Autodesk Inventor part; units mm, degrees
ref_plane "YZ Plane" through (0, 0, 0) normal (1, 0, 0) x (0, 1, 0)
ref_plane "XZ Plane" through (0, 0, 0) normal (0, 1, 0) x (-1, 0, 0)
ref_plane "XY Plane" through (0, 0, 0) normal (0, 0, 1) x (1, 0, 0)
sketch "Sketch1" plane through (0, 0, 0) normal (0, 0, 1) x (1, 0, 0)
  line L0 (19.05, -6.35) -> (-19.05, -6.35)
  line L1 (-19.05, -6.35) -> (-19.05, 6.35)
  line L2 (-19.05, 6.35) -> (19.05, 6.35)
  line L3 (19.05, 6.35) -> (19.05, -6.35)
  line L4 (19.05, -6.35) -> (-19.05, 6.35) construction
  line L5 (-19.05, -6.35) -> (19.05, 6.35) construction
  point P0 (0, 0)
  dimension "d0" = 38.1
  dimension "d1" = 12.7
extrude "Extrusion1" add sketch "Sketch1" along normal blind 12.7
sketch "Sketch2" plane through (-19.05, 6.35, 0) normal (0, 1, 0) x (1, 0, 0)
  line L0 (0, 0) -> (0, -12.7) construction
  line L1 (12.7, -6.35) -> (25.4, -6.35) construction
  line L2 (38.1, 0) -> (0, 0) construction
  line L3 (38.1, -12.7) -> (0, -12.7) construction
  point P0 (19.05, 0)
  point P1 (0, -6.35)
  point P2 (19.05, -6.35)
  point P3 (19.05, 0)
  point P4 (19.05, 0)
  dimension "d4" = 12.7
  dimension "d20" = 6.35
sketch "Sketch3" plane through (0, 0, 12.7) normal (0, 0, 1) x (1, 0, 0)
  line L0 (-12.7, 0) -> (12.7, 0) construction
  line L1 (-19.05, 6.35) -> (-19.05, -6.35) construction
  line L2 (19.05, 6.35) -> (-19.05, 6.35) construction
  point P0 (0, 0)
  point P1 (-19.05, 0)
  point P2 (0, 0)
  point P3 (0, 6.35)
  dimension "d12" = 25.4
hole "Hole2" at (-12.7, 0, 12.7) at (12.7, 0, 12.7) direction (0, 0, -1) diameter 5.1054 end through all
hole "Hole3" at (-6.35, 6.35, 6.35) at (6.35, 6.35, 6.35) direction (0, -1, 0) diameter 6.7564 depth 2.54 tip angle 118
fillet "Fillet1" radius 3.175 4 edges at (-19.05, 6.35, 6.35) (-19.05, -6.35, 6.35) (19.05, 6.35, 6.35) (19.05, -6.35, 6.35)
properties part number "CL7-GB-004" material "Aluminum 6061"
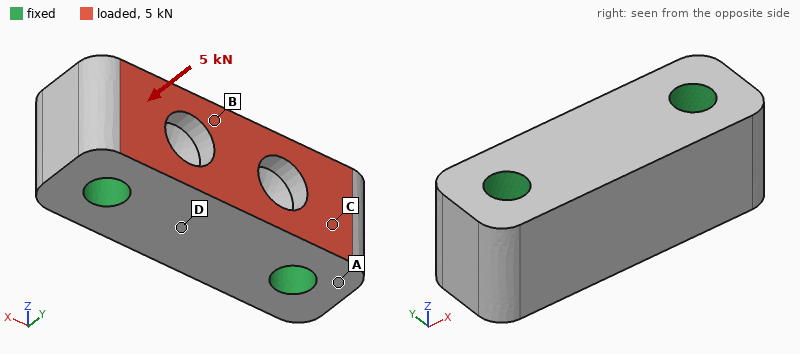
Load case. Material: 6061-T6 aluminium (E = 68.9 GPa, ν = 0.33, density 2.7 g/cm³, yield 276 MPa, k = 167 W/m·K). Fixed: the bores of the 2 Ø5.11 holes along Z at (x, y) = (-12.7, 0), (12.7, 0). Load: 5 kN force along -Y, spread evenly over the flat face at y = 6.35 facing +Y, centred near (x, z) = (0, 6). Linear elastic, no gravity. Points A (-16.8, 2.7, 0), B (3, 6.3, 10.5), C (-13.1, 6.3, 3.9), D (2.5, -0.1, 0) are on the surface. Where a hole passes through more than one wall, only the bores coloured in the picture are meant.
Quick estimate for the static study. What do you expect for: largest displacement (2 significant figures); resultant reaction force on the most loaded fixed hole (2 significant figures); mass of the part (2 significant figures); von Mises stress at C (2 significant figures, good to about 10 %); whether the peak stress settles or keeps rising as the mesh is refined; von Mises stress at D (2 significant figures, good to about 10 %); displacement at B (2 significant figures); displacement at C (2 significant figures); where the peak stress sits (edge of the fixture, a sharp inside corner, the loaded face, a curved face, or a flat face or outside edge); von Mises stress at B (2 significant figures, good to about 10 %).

5.3 µm
2.5 kN
14 g
18 MPa
keeps rising
9.6 MPa
4.8 µm
1.2 µm
edge of the fixture
21 MPa
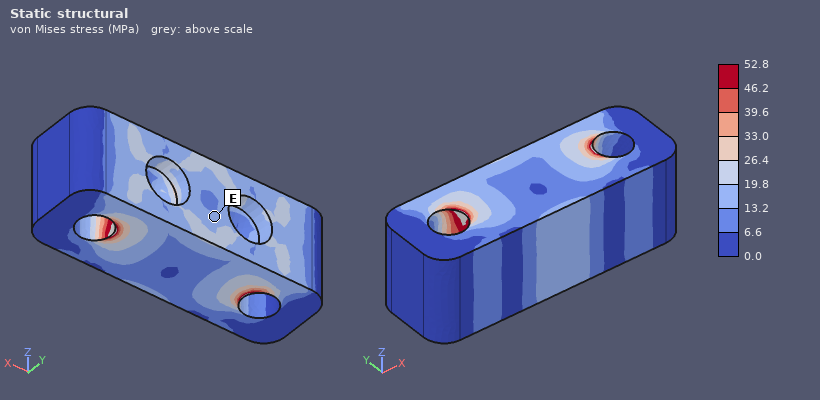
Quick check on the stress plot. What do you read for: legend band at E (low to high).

13.2 to 19.8 MPa
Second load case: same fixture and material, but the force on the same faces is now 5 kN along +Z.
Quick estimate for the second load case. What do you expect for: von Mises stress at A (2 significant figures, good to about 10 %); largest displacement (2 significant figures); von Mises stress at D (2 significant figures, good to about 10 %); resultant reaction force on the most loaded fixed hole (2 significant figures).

14 MPa
17 µm
31 MPa
2.5 kN
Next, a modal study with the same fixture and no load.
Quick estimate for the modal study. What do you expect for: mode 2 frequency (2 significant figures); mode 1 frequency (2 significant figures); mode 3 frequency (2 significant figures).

51 kHz
50 kHz
59 kHz
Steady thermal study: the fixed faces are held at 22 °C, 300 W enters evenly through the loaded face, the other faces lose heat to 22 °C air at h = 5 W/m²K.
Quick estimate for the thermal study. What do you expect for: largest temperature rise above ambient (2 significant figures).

50 K
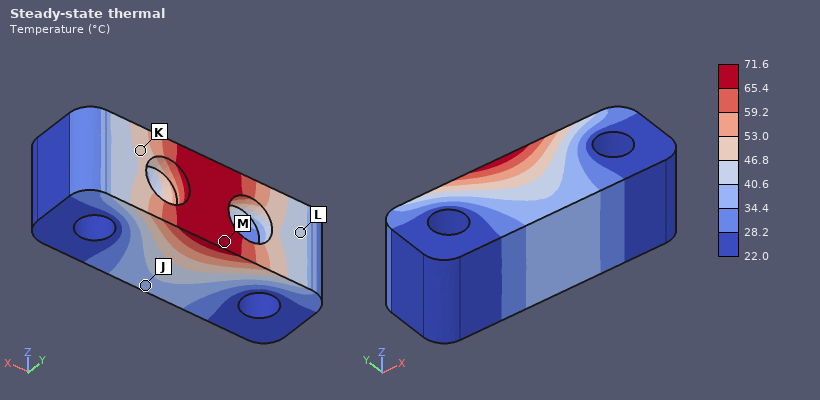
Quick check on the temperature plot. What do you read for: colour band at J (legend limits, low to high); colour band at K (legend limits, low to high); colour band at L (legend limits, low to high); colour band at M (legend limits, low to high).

34.4 to 40.6 °C
46.8 to 53.0 °C
40.6 to 46.8 °C
65.4 to 71.6 °C
